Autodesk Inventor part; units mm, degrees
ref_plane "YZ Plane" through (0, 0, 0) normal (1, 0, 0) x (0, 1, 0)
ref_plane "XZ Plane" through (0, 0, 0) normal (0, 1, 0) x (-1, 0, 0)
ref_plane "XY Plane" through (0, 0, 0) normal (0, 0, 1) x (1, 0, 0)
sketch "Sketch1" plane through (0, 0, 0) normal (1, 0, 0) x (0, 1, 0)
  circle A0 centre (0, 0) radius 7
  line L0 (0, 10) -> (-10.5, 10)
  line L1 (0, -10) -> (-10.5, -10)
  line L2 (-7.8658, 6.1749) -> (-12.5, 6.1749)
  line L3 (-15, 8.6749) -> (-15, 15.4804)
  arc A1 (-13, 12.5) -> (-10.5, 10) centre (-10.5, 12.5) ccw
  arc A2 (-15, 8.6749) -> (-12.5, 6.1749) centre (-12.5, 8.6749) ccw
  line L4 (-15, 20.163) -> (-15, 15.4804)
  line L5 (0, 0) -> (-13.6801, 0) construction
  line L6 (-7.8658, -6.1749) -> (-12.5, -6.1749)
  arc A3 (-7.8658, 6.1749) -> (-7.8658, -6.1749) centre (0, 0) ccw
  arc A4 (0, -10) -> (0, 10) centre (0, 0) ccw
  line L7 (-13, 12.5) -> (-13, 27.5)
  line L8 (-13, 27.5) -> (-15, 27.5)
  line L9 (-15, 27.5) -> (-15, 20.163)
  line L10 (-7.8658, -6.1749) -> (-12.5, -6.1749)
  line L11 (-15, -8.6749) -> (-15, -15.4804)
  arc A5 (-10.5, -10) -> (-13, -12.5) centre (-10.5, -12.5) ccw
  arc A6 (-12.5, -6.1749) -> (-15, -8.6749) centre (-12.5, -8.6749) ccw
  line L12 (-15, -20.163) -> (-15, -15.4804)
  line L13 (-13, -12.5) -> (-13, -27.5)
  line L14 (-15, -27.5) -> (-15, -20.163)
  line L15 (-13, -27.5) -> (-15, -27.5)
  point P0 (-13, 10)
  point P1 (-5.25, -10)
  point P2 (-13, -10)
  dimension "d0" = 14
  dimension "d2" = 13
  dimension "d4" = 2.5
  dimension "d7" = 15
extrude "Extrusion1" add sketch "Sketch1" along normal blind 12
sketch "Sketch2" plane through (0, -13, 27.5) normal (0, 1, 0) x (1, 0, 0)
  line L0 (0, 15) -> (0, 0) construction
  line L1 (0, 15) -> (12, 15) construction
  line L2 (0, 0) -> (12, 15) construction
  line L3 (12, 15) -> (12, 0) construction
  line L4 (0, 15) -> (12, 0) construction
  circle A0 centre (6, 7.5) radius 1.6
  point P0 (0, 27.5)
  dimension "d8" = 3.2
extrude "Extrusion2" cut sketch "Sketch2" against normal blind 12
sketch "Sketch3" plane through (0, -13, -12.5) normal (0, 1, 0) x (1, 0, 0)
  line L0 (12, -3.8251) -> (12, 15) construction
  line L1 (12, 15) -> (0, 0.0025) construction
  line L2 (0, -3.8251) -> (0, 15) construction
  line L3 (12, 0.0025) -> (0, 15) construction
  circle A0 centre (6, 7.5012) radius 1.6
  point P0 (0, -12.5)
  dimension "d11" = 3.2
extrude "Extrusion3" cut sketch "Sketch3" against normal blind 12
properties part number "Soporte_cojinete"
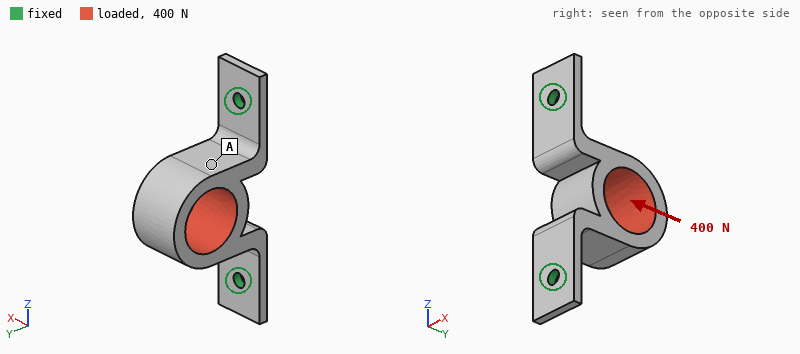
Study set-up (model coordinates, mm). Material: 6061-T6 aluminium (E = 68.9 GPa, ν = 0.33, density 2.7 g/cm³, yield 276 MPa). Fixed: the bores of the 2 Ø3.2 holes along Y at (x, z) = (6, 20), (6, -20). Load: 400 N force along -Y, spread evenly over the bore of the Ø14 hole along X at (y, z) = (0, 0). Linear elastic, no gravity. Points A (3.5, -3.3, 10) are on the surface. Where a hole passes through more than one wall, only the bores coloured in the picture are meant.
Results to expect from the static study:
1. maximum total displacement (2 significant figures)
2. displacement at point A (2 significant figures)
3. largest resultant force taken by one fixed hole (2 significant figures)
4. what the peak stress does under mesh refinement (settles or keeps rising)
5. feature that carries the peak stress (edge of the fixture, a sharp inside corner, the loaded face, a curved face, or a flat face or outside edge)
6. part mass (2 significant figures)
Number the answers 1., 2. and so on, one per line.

1. 31 µm
2. 30 µm
3. 280 N
4. keeps rising
5. edge of the fixture
6. 9.7 g
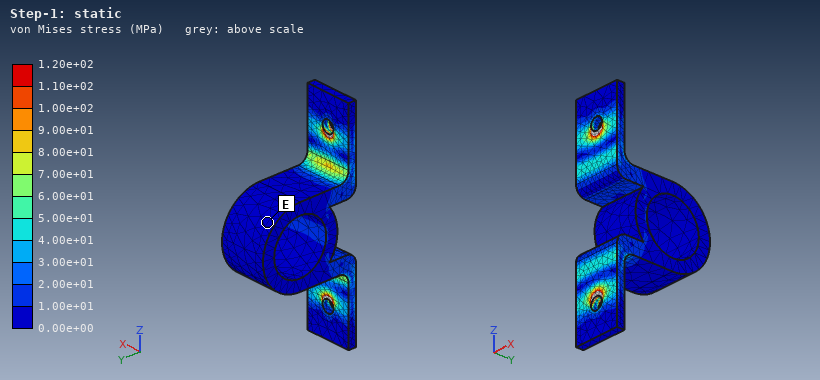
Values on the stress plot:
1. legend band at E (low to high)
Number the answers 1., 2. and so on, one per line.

1. 0.00e+00 to 1.00e+01 MPa
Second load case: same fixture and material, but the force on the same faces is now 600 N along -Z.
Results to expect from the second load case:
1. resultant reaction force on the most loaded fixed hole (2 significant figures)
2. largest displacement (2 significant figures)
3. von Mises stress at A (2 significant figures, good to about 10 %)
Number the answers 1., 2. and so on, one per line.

1. 400 N
2. 78 µm
3. 18 MPa
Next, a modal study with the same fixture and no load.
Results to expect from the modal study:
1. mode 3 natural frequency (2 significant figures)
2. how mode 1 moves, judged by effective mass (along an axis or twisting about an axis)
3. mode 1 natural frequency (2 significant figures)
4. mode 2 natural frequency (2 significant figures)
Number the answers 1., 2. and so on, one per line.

1. 6500 Hz
2. along X
3. 2000 Hz
4. 6300 Hz
